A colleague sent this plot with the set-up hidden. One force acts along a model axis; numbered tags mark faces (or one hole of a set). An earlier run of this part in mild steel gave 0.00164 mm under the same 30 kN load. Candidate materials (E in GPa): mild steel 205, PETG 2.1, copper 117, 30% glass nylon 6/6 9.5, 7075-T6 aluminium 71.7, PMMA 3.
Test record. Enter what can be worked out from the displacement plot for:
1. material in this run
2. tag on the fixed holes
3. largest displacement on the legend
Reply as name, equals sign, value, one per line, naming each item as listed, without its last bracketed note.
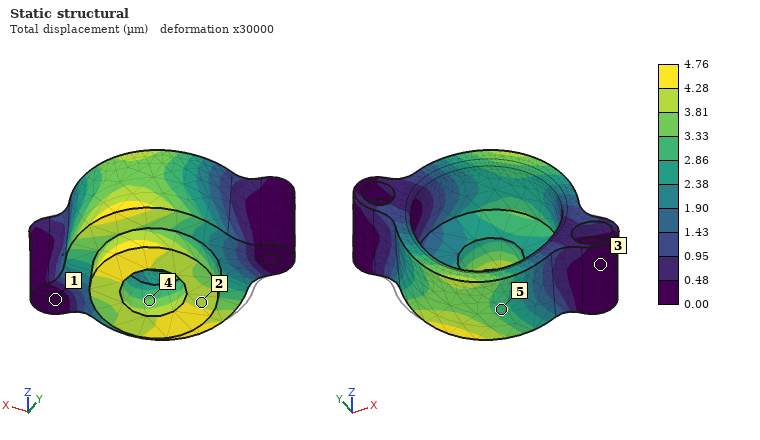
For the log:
material in this run = 7075-T6 aluminium
tag on the fixed holes = 1
largest displacement on the legend = 4.76 µm
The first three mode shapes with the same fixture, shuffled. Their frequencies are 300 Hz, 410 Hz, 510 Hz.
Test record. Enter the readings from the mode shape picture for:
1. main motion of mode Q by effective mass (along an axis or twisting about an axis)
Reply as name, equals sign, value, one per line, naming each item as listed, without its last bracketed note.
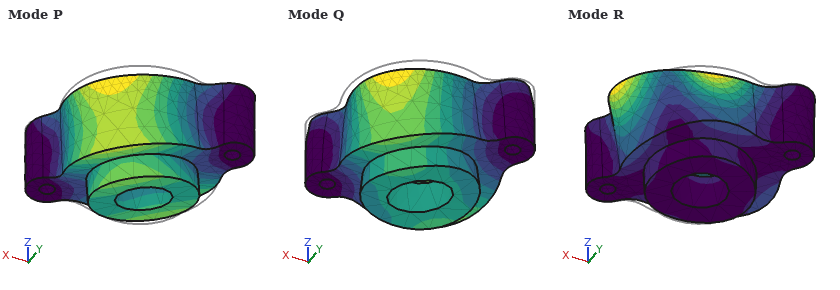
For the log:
main motion of mode Q by effective mass = along Z
